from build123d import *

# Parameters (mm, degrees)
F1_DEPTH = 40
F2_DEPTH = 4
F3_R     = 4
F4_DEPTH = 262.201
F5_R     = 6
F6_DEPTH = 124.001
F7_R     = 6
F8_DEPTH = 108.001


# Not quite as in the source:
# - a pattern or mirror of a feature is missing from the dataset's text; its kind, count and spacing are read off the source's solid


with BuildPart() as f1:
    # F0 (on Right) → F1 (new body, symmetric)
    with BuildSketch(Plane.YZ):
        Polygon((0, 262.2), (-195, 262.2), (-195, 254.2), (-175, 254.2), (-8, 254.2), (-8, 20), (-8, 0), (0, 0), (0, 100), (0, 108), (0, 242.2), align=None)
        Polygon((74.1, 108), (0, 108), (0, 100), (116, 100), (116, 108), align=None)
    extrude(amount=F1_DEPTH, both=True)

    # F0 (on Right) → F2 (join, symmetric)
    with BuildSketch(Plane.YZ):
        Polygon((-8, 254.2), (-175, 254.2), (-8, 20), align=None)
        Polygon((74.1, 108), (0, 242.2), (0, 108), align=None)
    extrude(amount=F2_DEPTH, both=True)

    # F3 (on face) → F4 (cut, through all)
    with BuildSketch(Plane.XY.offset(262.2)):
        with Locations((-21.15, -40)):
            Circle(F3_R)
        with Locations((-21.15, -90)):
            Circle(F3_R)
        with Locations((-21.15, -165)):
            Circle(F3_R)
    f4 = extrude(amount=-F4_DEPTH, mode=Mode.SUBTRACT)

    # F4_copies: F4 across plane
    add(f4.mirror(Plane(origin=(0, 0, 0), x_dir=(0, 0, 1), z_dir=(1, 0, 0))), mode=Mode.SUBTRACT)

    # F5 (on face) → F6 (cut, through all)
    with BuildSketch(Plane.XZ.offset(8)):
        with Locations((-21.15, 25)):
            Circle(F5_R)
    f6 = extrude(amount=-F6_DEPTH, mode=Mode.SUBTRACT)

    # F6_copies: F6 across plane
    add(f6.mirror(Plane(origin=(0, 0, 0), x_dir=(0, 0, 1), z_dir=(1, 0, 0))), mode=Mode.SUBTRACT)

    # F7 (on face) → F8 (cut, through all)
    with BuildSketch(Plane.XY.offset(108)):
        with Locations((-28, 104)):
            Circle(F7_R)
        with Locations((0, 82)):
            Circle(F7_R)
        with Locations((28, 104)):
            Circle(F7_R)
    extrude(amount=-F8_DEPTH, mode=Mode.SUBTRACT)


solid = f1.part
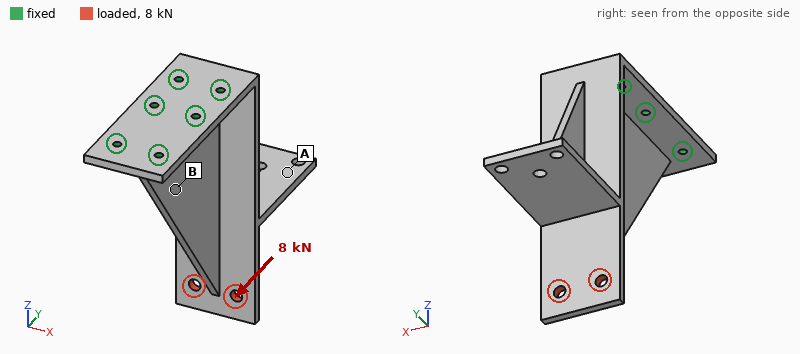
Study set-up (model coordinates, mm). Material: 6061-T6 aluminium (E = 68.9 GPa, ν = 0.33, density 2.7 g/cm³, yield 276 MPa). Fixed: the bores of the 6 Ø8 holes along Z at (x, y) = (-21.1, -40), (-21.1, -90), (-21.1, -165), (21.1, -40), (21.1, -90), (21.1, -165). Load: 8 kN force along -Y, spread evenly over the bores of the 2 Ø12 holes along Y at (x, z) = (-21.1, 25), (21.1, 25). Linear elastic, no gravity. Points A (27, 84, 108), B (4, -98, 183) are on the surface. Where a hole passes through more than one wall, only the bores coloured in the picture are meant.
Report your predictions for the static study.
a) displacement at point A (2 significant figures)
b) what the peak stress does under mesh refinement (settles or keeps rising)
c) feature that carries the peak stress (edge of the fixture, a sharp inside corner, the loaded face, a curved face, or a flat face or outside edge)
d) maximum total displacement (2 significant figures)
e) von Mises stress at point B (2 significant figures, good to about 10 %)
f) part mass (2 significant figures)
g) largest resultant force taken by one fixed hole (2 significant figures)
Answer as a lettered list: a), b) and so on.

a) 0.52 mm
b) keeps rising
c) edge of the fixture
d) 1.2 mm
e) 44 MPa
f) 1.5 kg
g) 8.7 kN
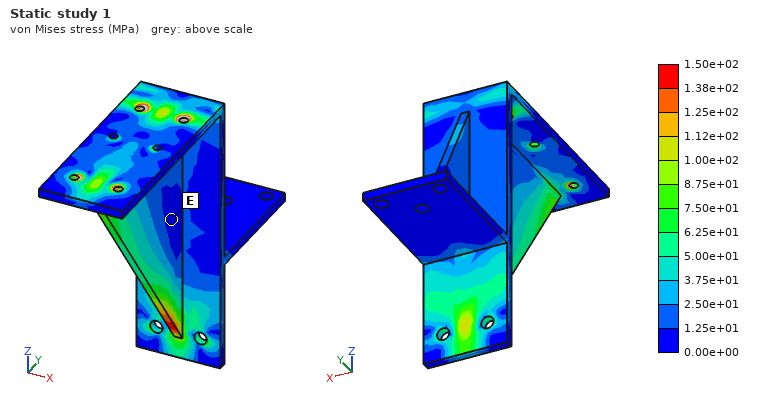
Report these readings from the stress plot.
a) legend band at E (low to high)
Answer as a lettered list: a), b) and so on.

a) 0.00e+00 to 1.25e+01 MPa
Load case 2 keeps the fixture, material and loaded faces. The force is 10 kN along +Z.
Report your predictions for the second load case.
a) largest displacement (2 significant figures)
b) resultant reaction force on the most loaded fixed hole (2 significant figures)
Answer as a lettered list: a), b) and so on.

a) 0.31 mm
b) 5.9 kN
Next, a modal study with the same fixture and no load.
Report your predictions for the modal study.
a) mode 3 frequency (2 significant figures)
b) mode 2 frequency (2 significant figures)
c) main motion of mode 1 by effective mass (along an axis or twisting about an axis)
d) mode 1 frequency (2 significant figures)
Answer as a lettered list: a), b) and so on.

a) 830 Hz
b) 420 Hz
c) along X
d) 210 Hz
